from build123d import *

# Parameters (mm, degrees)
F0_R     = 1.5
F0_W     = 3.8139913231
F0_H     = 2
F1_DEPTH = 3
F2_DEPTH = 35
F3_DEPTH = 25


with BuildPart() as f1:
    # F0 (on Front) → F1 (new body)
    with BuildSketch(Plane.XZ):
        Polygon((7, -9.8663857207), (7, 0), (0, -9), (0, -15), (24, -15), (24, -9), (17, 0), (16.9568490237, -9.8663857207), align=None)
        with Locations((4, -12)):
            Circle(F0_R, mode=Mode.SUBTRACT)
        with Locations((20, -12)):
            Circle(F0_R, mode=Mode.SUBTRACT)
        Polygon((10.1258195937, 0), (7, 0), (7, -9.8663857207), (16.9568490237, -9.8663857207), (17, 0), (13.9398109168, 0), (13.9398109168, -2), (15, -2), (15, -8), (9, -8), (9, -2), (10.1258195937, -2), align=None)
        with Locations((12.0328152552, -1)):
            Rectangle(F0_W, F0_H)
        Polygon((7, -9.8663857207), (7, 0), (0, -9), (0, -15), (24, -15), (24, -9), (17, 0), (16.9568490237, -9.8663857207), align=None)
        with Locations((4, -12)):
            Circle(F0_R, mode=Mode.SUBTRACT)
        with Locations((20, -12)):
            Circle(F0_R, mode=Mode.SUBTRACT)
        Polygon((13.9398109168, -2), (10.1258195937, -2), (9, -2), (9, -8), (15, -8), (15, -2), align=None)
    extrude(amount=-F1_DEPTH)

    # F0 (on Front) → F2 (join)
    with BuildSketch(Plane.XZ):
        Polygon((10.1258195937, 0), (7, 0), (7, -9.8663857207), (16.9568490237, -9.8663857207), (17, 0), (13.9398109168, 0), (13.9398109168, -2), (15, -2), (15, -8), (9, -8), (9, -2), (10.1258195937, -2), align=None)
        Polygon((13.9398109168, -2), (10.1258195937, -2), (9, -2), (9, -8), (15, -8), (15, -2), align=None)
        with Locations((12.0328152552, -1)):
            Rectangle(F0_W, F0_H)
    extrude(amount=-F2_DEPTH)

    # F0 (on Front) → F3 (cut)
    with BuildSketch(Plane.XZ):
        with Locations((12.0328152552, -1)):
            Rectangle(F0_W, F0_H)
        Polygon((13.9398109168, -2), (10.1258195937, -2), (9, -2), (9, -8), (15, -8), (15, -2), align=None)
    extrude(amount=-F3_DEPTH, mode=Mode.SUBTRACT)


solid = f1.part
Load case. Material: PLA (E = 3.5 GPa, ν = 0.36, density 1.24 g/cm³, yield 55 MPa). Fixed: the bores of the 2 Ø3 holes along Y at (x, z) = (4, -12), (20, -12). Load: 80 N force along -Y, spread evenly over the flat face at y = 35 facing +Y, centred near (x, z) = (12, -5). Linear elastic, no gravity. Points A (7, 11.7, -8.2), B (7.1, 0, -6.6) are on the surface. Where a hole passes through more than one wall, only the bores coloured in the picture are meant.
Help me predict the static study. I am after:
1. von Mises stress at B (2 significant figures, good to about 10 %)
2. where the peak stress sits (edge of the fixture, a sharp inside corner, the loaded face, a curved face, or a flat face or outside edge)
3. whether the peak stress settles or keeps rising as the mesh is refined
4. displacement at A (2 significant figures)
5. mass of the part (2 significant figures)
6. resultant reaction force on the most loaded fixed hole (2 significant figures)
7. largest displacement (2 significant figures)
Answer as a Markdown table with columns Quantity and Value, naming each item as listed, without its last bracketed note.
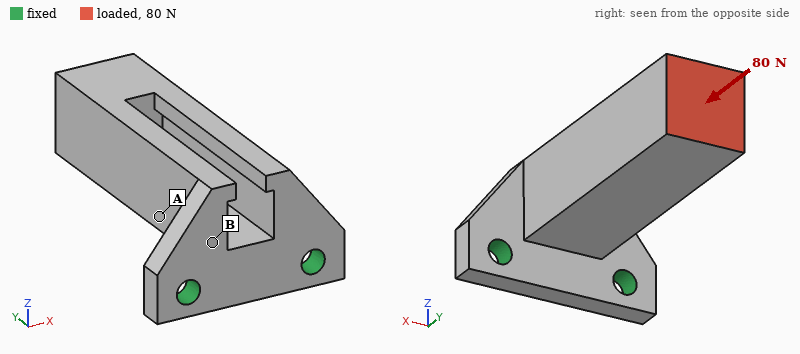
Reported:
| Quantity | Value |
|---|---|
| von Mises stress at B | 6.1 MPa |
| where the peak stress sits | edge of the fixture |
| whether the peak stress settles or keeps rising as the mesh is refined | keeps rising |
| displacement at A | 0.14 mm |
| mass of the part | 3.6 g |
| resultant reaction force on the most loaded fixed hole | 41 N |
| largest displacement | 0.48 mm |
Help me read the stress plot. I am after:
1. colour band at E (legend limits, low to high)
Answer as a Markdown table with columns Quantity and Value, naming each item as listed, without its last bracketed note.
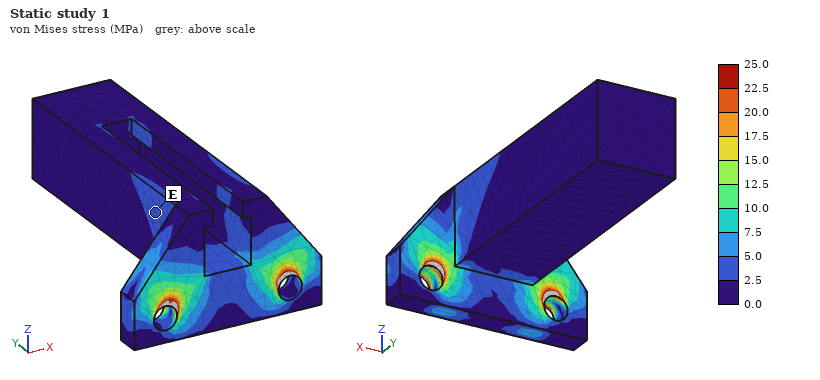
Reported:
| Quantity | Value |
|---|---|
| colour band at E | 2.5 to 5.0 MPa |
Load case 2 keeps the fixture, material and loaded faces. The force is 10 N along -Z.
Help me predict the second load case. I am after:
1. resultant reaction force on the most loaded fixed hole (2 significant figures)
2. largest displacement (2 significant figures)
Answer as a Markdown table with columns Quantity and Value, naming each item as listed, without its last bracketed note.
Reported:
| Quantity | Value |
|---|---|
| resultant reaction force on the most loaded fixed hole | 5.6 N |
| largest displacement | 0.46 mm |
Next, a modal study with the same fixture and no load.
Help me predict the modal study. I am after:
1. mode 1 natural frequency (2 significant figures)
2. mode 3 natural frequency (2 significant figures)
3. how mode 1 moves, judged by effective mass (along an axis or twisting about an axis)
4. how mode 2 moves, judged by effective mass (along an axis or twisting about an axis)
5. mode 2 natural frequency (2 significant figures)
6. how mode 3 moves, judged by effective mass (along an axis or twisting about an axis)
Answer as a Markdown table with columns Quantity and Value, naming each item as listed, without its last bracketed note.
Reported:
| Quantity | Value |
|---|---|
| mode 1 natural frequency | 700 Hz |
| mode 3 natural frequency | 2600 Hz |
| how mode 1 moves, judged by effective mass | along Z |
| how mode 2 moves, judged by effective mass | along X |
| mode 2 natural frequency | 1200 Hz |
| how mode 3 moves, judged by effective mass | twisting about Y |
